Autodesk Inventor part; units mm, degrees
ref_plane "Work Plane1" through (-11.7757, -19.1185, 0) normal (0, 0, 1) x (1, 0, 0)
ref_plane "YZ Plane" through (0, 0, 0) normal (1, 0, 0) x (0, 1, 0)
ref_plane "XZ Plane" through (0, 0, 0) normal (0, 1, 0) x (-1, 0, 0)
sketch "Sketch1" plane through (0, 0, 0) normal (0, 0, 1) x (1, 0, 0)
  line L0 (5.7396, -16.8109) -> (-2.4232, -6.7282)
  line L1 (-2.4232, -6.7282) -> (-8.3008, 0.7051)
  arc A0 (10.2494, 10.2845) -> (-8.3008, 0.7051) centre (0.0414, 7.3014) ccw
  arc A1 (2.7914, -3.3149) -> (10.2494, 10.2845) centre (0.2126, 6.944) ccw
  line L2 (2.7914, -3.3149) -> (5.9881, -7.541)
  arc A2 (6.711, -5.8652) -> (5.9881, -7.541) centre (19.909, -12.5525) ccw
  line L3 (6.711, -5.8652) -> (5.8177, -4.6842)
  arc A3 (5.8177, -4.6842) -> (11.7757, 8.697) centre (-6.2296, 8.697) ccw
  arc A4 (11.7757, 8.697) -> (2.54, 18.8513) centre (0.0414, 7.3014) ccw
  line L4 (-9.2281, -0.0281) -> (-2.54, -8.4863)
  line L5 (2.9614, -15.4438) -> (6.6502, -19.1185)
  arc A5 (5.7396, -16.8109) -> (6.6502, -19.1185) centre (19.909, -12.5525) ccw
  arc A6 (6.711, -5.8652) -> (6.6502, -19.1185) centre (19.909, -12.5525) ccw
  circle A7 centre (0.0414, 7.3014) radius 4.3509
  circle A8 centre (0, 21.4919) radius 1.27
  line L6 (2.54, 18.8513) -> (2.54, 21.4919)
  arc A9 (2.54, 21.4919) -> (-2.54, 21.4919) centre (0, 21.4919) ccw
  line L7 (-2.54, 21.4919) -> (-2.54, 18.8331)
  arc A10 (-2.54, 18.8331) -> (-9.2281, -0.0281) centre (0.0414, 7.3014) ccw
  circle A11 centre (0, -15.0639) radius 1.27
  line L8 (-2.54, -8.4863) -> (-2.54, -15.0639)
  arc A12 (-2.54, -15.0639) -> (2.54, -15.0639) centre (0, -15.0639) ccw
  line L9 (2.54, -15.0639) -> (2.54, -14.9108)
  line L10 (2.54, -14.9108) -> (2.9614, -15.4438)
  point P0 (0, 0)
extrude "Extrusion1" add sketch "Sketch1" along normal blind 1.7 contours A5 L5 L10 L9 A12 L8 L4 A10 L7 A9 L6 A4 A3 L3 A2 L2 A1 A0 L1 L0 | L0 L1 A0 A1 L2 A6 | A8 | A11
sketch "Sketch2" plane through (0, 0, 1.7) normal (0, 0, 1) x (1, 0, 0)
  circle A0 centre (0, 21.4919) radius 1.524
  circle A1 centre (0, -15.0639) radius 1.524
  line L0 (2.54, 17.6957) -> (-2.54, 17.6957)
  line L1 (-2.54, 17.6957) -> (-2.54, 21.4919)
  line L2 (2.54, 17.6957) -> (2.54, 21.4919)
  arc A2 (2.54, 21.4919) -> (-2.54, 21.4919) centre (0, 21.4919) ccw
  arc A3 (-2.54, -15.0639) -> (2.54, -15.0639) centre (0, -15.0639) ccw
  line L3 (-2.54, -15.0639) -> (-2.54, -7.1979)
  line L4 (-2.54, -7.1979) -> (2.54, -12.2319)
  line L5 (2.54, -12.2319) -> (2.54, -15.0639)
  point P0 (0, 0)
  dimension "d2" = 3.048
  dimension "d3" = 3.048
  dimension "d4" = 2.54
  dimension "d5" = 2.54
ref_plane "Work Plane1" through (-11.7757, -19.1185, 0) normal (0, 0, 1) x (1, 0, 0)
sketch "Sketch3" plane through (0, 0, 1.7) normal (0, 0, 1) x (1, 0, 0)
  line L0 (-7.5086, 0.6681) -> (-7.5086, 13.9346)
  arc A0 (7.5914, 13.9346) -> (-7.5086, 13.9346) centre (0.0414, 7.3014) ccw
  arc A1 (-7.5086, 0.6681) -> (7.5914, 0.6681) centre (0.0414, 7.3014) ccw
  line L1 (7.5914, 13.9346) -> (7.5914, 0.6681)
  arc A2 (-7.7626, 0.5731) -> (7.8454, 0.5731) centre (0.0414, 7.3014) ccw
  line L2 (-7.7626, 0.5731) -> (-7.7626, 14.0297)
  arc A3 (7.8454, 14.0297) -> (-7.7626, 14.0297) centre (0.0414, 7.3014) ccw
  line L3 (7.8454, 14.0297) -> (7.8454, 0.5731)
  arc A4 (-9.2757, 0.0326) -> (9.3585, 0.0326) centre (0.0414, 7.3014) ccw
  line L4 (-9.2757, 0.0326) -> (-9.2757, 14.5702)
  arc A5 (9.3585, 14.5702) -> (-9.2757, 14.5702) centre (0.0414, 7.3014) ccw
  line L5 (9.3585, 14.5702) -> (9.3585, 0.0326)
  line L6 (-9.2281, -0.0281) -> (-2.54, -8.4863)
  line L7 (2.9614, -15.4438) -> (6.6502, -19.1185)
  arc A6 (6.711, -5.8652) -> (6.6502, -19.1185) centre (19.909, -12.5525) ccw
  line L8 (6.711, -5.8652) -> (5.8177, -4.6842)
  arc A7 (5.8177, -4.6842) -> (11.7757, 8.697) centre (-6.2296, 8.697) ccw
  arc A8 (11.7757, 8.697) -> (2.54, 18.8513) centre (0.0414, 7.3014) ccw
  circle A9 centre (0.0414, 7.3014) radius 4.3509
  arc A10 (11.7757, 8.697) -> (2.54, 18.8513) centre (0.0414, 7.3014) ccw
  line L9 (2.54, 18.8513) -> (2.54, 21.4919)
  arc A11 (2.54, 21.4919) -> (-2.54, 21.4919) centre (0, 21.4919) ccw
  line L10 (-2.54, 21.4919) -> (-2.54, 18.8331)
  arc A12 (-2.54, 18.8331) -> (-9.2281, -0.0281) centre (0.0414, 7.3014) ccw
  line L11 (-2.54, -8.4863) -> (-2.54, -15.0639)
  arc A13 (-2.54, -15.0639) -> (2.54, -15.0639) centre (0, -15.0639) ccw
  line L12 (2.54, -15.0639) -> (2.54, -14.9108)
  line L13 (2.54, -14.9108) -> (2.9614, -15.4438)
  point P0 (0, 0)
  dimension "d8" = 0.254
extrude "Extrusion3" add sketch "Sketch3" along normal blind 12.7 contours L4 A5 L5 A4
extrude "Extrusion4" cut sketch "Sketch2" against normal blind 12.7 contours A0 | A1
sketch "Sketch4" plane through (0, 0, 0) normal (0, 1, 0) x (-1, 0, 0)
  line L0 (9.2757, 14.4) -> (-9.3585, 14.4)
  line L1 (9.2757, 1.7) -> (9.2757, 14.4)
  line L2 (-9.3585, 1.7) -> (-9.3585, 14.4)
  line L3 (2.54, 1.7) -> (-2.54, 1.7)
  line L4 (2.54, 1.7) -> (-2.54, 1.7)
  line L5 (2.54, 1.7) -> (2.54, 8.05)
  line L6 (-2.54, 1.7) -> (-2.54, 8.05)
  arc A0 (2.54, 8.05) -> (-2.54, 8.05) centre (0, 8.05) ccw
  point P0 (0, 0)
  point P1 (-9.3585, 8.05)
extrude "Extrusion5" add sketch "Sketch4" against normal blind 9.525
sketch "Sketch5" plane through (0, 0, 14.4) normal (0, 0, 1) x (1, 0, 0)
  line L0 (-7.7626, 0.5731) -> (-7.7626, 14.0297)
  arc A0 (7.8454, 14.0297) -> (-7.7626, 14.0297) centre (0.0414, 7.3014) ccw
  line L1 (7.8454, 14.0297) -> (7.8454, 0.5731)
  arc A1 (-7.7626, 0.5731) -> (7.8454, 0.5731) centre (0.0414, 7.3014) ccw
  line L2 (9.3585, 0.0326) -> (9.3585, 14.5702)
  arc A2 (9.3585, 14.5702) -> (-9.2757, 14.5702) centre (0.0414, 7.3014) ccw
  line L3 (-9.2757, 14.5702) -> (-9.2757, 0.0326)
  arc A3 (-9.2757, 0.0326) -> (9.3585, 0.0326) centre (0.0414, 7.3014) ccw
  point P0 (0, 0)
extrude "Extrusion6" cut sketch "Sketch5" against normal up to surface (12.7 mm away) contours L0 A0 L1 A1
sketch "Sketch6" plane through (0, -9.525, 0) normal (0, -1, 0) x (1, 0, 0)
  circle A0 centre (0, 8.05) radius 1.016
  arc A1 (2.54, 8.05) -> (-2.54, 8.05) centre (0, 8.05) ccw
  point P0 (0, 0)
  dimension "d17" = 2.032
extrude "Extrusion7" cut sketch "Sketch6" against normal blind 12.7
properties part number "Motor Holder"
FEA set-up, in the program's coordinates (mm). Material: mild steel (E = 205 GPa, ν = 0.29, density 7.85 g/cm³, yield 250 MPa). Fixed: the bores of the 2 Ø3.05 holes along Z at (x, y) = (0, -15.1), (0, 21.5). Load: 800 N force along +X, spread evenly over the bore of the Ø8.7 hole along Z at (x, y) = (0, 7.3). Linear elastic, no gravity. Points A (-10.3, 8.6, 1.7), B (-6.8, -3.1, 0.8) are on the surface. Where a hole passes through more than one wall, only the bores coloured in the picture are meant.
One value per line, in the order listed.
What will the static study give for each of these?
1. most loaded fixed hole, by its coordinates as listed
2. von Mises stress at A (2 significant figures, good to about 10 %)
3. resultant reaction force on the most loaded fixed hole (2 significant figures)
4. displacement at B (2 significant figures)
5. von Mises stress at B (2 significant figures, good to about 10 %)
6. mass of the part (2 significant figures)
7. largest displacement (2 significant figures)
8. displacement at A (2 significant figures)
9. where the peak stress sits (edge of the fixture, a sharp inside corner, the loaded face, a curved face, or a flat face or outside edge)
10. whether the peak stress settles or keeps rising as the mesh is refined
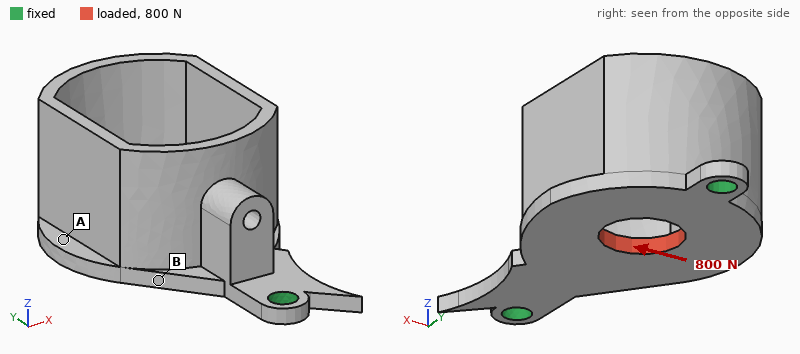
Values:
(0, 21.5)
17 MPa
490 N
6.2 µm
45 MPa
18 g
7.1 µm
5.4 µm
edge of the fixture
keeps rising
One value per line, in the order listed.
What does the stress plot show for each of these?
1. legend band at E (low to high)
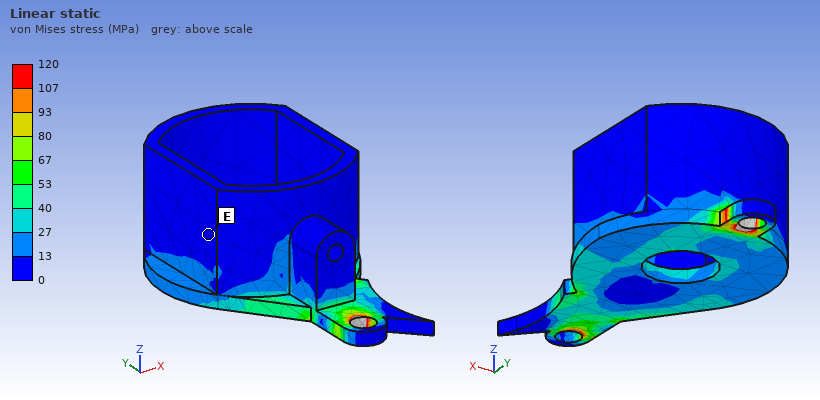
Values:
0 to 13 MPa
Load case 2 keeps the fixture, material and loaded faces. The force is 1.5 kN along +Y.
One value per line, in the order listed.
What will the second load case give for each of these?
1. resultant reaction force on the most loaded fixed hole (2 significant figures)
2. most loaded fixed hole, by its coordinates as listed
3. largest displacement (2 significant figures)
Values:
840 N
(0, 21.5)
4.5 µm
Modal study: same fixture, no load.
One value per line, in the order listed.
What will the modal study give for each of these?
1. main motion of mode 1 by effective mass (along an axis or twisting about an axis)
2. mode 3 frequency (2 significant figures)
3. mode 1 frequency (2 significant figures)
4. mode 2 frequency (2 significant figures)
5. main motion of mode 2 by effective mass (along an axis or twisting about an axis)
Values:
along X
11 kHz
3200 Hz
7700 Hz
along Z
